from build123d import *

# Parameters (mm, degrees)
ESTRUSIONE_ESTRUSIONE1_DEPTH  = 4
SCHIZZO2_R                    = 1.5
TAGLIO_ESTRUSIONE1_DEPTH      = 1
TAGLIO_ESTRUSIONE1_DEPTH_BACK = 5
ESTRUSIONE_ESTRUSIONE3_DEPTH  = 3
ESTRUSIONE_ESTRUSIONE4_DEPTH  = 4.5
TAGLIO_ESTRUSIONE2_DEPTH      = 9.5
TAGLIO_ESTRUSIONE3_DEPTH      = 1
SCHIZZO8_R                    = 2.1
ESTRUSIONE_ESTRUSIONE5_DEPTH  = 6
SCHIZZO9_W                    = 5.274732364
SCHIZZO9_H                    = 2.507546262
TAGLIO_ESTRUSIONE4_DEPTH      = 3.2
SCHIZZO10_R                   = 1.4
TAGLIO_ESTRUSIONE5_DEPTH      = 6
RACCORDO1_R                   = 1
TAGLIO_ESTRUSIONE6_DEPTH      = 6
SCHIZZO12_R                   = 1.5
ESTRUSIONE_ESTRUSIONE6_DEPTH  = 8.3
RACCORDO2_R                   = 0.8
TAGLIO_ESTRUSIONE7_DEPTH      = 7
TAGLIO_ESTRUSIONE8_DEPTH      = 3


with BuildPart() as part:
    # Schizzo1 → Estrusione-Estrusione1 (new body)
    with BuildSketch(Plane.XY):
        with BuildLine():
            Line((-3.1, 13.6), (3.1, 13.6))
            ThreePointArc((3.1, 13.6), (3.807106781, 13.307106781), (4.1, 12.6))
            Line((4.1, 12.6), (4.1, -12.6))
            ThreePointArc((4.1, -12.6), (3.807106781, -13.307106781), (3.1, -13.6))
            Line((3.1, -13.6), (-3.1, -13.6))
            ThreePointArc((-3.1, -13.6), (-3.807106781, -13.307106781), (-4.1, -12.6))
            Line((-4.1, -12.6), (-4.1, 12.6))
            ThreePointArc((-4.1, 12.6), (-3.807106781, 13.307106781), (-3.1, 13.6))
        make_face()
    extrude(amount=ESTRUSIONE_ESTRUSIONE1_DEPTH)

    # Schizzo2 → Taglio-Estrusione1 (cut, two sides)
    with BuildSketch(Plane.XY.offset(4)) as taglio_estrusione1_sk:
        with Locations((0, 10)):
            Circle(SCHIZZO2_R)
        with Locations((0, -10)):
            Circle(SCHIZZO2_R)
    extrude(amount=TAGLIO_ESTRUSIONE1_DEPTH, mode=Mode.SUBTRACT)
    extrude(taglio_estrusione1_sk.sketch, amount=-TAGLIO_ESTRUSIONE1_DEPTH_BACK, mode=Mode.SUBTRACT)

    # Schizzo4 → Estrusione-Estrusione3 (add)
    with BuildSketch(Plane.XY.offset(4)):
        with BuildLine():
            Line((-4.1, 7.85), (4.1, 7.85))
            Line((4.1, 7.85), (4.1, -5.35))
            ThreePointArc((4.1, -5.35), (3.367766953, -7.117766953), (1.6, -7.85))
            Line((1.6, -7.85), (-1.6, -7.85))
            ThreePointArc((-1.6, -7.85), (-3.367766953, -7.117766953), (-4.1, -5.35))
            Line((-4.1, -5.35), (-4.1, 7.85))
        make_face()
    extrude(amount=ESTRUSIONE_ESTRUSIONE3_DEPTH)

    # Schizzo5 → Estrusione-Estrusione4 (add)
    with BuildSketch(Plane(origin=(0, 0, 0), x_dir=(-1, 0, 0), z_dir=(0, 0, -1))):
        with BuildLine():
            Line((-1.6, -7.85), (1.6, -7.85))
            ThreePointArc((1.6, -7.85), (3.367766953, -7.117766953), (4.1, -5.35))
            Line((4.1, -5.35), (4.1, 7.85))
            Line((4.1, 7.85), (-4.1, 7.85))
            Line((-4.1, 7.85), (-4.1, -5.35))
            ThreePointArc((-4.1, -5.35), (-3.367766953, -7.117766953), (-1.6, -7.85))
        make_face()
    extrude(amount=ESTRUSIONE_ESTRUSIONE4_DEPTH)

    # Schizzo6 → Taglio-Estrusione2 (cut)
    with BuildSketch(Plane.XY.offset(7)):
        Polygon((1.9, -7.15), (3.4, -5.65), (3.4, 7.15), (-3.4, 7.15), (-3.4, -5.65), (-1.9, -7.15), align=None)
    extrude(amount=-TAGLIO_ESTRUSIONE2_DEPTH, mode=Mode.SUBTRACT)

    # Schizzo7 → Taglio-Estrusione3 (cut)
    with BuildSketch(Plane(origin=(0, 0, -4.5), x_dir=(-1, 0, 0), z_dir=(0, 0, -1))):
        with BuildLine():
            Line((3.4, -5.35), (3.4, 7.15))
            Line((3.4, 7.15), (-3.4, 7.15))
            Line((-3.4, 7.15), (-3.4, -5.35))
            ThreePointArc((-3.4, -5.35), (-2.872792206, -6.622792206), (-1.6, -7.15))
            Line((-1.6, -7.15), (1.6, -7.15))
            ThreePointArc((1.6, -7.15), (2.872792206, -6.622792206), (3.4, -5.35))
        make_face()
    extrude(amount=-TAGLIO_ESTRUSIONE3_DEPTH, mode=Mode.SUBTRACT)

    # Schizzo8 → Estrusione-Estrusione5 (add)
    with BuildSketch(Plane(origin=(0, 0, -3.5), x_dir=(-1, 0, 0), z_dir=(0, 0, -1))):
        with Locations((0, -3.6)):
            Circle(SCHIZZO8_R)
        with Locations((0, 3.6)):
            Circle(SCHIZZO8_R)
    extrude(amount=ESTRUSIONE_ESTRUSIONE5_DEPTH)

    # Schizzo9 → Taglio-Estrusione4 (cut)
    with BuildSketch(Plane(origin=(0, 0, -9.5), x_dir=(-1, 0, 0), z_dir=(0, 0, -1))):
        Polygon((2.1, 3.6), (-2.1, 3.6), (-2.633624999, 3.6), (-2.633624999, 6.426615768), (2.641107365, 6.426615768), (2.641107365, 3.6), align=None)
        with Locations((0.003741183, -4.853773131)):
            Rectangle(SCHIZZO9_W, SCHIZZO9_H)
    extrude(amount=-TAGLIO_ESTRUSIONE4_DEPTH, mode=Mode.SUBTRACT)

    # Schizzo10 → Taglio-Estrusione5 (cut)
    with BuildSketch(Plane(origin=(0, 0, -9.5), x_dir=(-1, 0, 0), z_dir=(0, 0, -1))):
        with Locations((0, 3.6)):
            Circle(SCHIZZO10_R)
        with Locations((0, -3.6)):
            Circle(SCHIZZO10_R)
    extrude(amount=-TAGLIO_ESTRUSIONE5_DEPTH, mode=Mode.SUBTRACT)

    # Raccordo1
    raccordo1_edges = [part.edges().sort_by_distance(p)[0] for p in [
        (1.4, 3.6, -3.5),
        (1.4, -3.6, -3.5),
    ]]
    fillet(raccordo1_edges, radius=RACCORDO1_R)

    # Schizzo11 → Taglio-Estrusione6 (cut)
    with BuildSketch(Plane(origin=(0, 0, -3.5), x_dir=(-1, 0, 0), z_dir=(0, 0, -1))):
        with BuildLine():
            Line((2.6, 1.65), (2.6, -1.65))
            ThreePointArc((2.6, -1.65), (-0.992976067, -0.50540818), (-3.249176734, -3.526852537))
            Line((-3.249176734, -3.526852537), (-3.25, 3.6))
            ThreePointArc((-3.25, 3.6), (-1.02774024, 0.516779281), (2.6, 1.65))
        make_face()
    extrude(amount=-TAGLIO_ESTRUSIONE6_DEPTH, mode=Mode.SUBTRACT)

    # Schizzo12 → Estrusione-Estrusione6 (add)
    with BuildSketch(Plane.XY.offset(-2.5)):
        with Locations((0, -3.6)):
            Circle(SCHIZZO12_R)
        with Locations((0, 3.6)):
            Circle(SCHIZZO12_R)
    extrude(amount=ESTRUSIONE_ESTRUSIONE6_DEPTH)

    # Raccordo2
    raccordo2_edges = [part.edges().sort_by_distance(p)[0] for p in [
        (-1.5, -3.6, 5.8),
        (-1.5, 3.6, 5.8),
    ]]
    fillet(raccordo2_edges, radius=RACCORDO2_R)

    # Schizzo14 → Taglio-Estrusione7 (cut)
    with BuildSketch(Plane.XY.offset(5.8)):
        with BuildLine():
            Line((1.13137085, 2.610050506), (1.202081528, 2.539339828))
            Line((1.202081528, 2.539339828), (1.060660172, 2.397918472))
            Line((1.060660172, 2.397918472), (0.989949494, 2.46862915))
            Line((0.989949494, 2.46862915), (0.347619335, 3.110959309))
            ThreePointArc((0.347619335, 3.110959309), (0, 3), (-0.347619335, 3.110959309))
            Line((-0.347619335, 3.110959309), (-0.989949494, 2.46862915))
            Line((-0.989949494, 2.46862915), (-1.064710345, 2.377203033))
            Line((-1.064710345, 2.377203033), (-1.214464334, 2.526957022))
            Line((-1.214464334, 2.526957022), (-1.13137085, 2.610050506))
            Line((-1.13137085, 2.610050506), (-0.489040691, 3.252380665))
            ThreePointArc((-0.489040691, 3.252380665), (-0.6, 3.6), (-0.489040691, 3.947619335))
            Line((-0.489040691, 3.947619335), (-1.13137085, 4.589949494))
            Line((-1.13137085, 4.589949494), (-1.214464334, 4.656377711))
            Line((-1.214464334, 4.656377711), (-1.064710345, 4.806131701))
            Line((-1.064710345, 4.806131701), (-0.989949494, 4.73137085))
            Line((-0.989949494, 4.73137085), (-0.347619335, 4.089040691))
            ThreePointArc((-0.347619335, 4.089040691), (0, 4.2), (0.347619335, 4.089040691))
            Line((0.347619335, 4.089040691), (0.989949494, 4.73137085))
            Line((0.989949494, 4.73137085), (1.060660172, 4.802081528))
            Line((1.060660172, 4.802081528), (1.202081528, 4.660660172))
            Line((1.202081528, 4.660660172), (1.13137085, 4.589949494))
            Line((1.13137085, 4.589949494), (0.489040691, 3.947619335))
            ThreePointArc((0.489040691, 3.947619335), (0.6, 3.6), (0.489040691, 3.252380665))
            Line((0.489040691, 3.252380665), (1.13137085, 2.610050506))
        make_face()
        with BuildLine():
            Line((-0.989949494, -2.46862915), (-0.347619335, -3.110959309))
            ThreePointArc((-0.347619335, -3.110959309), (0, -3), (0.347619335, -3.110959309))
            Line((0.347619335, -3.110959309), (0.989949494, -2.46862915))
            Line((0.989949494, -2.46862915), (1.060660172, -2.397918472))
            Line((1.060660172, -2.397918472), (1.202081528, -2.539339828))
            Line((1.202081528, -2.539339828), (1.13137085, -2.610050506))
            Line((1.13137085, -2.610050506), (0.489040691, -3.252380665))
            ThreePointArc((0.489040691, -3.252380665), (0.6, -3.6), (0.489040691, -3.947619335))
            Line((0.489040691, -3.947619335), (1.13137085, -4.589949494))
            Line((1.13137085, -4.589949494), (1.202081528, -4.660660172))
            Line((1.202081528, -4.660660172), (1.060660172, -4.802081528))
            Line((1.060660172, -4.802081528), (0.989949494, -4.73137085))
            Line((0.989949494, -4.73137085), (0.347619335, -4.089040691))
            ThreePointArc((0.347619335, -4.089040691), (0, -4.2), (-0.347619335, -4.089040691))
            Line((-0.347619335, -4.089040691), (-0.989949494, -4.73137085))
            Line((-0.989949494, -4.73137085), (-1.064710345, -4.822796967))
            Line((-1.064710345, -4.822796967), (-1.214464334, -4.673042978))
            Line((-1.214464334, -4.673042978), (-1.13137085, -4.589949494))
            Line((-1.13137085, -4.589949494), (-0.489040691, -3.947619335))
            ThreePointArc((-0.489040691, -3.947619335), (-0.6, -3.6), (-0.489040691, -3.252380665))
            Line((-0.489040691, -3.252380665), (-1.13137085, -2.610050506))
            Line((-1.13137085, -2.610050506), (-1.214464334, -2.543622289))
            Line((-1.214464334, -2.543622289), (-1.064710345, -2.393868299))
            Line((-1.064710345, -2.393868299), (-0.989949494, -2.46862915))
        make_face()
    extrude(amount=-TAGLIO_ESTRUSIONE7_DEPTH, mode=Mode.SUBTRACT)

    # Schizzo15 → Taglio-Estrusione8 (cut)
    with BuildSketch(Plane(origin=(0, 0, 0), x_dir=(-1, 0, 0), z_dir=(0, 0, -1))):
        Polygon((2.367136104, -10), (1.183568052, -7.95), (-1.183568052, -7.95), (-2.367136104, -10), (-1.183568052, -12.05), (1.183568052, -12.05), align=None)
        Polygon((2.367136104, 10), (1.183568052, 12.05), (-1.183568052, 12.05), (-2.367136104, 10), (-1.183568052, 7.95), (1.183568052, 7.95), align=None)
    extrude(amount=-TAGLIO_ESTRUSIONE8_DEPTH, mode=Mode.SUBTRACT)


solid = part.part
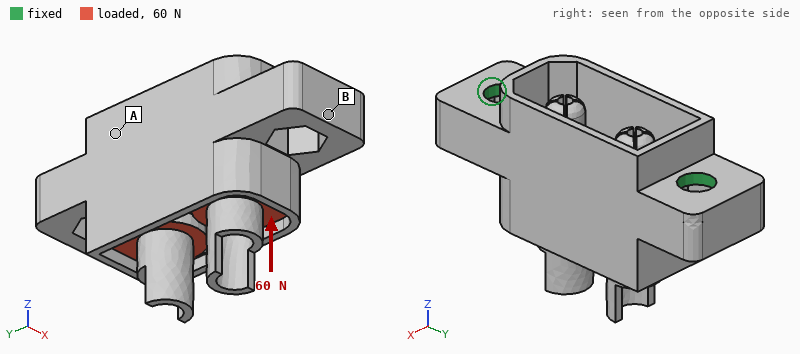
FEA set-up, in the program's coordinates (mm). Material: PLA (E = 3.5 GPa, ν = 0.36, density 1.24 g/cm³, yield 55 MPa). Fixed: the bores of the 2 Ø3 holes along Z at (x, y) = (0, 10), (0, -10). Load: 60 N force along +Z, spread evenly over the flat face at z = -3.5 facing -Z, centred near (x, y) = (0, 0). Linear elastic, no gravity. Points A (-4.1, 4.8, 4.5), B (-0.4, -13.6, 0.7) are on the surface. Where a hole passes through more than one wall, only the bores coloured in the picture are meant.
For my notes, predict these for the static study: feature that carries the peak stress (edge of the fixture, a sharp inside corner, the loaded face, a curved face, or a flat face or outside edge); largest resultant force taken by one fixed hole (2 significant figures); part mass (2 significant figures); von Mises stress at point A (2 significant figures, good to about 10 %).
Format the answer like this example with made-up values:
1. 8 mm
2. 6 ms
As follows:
1. a flat face or outside edge
2. 32 N
3. 1.1 g
4. 2.8 MPa
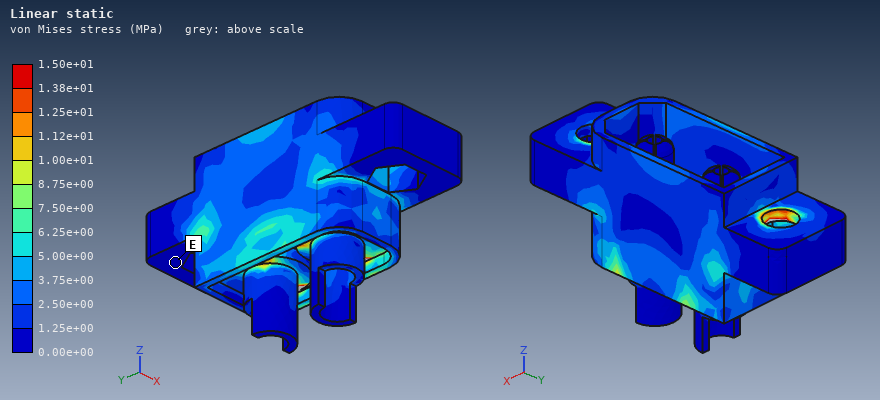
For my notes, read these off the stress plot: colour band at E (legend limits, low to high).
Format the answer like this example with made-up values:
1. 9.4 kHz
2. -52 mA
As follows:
1. 0.00e+00 to 1.25e+00 MPa
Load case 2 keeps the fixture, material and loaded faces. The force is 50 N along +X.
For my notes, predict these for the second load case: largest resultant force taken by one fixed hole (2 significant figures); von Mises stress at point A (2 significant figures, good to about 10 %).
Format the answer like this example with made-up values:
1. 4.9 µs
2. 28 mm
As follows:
1. 25 N
2. 2.8 MPa
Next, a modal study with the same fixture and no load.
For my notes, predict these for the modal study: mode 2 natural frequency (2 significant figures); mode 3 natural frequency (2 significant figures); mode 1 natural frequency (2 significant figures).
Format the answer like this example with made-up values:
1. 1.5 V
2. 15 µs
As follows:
1. 3900 Hz
2. 4100 Hz
3. 3900 Hz
